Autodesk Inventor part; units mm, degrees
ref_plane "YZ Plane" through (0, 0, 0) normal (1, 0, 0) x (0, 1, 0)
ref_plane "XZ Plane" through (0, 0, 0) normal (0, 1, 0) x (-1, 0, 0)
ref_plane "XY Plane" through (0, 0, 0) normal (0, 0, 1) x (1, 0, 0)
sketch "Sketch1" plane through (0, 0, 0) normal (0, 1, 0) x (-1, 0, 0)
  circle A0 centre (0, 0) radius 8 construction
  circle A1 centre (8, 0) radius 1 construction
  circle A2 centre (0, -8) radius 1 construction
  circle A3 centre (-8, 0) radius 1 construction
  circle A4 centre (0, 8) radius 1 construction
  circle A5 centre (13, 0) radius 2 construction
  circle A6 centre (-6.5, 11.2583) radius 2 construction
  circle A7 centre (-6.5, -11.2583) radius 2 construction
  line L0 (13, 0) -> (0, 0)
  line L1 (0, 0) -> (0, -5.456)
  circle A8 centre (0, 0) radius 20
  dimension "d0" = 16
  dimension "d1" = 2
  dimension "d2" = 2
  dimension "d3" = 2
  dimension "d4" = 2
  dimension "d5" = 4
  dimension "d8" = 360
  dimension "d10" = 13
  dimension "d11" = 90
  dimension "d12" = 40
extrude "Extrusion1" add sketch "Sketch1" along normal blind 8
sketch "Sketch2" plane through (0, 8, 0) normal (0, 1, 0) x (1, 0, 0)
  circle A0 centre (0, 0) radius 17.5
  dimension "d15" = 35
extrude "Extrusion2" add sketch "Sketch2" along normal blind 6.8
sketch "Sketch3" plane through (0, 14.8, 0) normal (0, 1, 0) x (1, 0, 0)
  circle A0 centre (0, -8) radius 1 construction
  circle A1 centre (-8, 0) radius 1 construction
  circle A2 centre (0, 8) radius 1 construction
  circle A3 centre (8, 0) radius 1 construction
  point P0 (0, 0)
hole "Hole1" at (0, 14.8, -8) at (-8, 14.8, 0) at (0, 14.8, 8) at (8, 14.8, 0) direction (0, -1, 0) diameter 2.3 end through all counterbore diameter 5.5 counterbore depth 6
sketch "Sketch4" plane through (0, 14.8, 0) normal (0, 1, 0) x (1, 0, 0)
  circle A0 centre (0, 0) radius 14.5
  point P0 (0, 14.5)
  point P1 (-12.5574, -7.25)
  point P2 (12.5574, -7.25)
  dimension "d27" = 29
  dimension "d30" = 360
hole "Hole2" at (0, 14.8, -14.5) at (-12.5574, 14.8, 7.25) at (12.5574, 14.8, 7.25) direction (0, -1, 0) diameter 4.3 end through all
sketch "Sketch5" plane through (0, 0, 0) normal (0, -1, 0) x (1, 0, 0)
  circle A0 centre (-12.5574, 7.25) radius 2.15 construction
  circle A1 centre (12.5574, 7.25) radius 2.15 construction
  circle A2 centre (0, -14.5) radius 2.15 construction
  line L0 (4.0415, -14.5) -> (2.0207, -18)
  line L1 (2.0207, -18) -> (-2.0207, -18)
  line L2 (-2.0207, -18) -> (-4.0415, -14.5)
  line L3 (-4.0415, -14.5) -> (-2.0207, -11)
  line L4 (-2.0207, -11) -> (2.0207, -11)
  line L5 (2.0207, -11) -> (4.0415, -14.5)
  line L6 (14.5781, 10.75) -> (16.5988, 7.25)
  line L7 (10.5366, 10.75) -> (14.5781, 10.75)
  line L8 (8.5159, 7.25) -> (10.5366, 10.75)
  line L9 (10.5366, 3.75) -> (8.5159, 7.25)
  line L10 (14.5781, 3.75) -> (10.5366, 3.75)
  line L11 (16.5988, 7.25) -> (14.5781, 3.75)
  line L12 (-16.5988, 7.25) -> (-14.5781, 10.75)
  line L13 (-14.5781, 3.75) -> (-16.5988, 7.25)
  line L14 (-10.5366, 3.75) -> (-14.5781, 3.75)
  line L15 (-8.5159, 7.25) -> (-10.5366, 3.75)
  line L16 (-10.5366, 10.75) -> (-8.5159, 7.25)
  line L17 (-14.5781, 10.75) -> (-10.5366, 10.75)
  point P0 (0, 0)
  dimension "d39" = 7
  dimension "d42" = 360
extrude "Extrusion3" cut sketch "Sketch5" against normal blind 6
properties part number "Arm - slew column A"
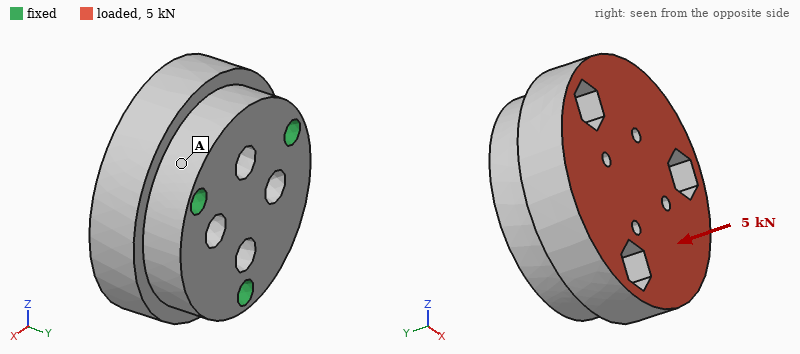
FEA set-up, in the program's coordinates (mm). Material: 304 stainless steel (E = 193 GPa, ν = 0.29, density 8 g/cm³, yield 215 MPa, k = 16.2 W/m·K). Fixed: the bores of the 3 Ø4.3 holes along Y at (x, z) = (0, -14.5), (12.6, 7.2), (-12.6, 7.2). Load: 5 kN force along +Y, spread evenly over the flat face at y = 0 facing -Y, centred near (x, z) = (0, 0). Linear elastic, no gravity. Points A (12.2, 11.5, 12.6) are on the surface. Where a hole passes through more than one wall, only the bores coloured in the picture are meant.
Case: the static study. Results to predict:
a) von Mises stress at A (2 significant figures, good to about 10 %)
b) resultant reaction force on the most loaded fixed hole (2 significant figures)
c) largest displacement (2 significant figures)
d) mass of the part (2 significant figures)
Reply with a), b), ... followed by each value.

a) 12 MPa
b) 1.7 kN
c) 1.7 µm
d) 120 g
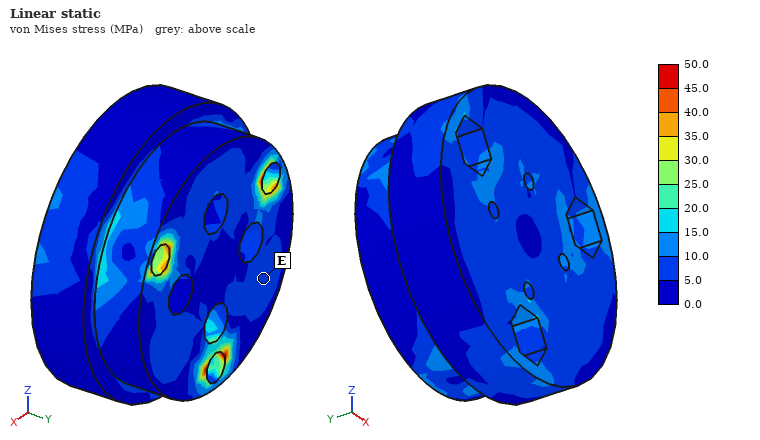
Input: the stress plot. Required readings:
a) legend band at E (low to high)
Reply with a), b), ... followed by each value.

a) 5.0 to 10.0 MPa
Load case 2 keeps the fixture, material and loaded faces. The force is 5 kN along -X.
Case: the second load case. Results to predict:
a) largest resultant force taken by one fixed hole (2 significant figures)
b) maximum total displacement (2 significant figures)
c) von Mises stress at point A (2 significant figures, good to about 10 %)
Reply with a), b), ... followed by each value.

a) 2.3 kN
b) 3.9 µm
c) 11 MPa
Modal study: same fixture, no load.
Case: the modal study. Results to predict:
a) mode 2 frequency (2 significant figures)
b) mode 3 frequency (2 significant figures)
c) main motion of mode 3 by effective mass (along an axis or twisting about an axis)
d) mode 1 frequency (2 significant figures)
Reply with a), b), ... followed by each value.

a) 28 kHz
b) 34 kHz
c) along Y
d) 28 kHz
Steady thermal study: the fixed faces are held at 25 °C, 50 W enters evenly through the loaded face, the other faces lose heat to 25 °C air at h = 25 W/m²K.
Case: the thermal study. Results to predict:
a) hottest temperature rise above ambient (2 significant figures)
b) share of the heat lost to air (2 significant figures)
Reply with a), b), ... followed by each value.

a) 55 K
b) 6.1 %
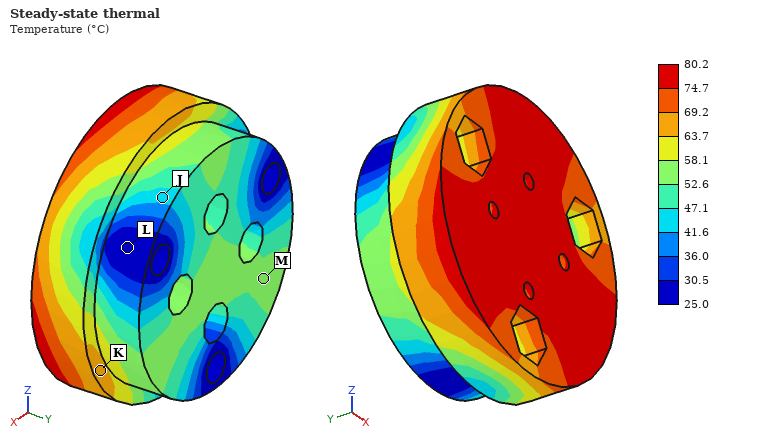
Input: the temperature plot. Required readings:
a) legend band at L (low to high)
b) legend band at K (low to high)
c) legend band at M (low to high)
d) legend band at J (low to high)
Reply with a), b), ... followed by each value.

a) 25.0 to 30.5 °C
b) 63.7 to 69.2 °C
c) 52.6 to 58.1 °C
d) 41.6 to 47.1 °C
